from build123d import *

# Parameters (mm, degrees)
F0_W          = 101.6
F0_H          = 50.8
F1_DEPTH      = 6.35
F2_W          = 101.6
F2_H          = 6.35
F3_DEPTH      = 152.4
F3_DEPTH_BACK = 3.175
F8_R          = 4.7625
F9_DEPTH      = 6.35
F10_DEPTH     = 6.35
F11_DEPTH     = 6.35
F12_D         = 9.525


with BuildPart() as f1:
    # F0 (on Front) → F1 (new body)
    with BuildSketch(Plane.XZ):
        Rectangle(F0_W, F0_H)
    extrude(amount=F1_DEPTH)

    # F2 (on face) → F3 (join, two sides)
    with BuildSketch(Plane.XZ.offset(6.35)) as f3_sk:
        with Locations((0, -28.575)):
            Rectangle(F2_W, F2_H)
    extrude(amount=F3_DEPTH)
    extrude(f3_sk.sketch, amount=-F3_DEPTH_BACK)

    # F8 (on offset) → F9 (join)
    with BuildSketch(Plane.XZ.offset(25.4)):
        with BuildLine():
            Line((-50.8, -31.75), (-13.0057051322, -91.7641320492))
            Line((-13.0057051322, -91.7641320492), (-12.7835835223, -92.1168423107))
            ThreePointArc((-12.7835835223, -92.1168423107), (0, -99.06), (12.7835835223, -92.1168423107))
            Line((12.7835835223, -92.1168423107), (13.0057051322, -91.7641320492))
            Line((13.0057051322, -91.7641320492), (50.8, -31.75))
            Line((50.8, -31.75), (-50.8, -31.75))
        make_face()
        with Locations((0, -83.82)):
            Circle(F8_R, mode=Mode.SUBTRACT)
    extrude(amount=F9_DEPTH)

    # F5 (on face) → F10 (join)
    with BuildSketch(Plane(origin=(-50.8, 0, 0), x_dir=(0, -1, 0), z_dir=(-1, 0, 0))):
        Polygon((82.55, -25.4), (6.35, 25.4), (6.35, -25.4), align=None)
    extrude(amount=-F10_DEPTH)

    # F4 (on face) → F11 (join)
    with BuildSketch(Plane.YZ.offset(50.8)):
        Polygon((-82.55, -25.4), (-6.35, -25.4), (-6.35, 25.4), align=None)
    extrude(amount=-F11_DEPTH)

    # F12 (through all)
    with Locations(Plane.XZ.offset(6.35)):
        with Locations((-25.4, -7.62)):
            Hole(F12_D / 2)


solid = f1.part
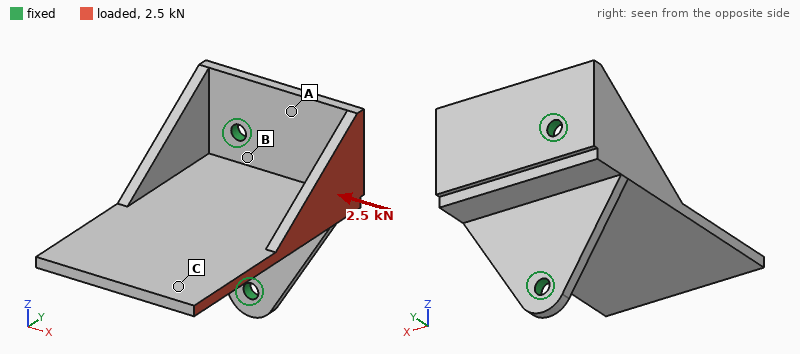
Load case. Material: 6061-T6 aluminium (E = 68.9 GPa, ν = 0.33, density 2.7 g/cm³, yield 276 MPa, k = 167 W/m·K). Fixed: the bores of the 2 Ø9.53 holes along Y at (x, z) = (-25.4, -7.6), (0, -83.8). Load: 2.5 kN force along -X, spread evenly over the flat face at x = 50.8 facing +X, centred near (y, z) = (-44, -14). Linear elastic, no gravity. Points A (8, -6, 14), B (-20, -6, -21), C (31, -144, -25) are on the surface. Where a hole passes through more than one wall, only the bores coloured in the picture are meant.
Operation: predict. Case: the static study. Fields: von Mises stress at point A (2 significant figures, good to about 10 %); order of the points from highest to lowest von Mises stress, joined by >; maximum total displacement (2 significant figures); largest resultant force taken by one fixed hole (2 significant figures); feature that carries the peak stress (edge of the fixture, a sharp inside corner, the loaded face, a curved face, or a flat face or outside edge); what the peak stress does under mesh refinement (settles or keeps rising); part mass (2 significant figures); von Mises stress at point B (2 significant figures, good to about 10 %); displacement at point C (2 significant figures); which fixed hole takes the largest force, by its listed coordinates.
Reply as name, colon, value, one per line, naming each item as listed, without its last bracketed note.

von Mises stress at point A: 23 MPa
order of the points from highest to lowest von Mises stress, joined by >: B > A > C
maximum total displacement: 0.73 mm
largest resultant force taken by one fixed hole: 1.5 kN
feature that carries the peak stress: edge of the fixture
what the peak stress does under mesh refinement: keeps rising
part mass: 490 g
von Mises stress at point B: 37 MPa
displacement at point C: 0.63 mm
which fixed hole takes the largest force, by its listed coordinates: (0, -83.8)
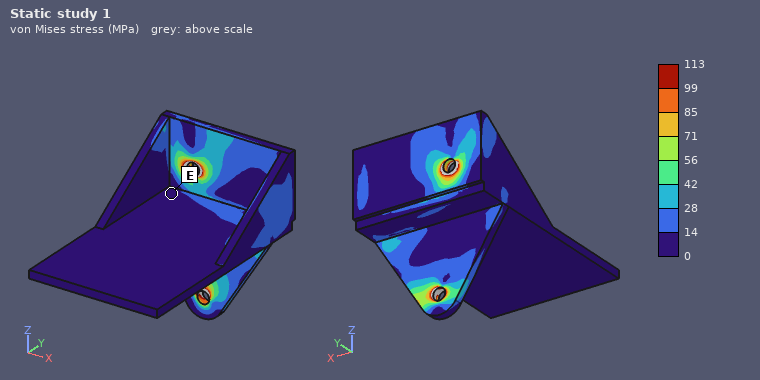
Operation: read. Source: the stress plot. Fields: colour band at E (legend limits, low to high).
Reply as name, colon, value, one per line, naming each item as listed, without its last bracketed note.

colour band at E: 0 to 14 MPa
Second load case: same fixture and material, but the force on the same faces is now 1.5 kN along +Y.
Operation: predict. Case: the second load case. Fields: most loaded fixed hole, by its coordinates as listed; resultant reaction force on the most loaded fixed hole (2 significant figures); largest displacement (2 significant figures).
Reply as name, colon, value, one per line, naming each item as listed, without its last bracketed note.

most loaded fixed hole, by its coordinates as listed: (-25.4, -7.6)
resultant reaction force on the most loaded fixed hole: 1.9 kN
largest displacement: 0.82 mm
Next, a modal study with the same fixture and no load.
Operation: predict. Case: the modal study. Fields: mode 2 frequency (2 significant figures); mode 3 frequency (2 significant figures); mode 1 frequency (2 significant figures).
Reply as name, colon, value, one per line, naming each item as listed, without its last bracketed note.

mode 2 frequency: 510 Hz
mode 3 frequency: 1100 Hz
mode 1 frequency: 420 Hz
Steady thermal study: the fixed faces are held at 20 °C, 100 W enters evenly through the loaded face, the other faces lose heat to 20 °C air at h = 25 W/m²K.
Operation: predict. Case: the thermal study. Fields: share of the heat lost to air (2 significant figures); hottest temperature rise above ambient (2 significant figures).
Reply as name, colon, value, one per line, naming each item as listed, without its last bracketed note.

share of the heat lost to air: 33 %
hottest temperature rise above ambient: 50 K
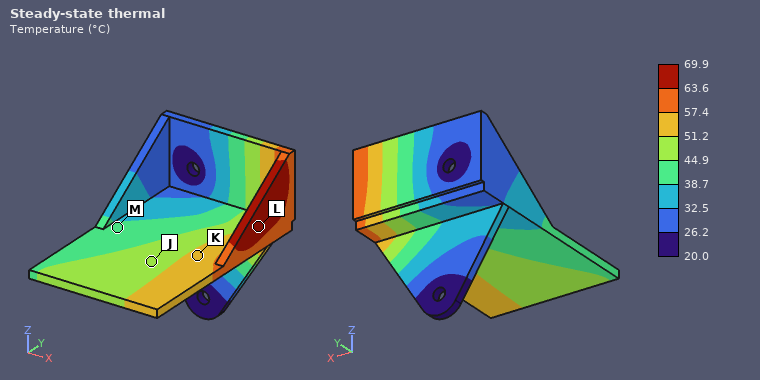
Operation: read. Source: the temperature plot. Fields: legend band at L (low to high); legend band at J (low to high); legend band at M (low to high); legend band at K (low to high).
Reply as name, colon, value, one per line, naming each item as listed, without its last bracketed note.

legend band at L: 63.6 to 69.9 °C
legend band at J: 44.9 to 51.2 °C
legend band at M: 38.7 to 44.9 °C
legend band at K: 51.2 to 57.4 °C
